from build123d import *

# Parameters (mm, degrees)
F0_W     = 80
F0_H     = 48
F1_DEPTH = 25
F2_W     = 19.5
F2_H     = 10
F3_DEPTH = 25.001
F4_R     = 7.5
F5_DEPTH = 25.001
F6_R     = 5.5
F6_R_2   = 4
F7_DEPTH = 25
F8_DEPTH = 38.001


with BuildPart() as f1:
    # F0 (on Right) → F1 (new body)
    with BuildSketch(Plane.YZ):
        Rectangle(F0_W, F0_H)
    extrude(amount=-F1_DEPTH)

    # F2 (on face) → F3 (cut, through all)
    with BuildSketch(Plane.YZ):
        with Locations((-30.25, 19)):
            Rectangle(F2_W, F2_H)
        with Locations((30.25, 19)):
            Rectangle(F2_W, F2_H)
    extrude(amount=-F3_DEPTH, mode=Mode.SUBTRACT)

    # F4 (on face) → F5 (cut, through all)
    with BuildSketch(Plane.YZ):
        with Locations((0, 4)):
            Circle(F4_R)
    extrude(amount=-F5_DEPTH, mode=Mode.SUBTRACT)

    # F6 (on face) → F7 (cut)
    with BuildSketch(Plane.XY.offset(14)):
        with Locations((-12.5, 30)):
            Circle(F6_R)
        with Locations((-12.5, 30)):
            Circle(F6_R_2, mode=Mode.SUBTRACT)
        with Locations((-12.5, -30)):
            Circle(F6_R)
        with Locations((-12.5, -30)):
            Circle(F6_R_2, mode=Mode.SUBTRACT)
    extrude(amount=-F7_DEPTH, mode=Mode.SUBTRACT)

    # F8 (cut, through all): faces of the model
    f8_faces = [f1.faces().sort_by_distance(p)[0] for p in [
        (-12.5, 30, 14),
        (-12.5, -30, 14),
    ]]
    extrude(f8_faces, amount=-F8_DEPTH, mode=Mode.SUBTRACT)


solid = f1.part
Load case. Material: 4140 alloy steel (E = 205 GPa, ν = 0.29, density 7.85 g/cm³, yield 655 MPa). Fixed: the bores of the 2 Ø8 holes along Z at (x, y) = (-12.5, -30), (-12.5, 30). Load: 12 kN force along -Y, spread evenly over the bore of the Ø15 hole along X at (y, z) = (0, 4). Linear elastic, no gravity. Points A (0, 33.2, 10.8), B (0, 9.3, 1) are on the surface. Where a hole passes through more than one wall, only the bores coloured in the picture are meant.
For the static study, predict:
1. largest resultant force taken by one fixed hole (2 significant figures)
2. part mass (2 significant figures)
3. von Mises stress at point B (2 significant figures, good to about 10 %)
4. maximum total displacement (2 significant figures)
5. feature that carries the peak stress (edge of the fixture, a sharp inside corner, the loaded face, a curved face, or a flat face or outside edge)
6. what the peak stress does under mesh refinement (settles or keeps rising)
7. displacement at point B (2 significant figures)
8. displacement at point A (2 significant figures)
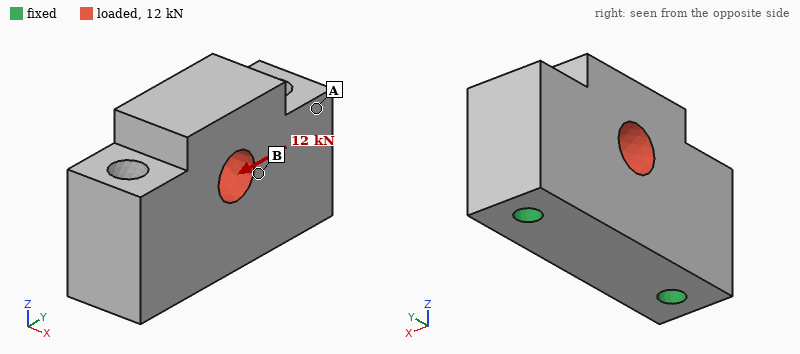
7.1 kN
590 g
14 MPa
4.7 µm
edge of the fixture
keeps rising
3.0 µm
3.7 µm
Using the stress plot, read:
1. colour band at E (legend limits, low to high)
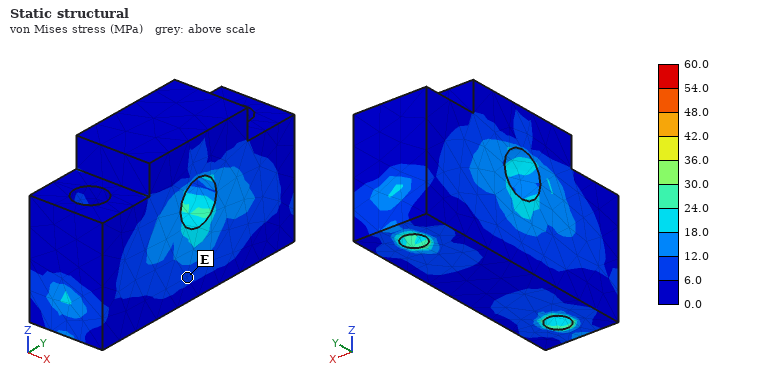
6.0 to 12.0 MPa
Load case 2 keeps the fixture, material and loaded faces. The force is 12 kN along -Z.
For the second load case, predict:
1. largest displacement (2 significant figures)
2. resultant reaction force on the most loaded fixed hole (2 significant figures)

4.0 µm
6.5 kN
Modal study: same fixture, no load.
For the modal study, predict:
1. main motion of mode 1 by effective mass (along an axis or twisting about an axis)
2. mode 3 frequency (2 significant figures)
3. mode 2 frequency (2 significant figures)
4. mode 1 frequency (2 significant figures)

along X
14 kHz
14 kHz
5800 Hz
